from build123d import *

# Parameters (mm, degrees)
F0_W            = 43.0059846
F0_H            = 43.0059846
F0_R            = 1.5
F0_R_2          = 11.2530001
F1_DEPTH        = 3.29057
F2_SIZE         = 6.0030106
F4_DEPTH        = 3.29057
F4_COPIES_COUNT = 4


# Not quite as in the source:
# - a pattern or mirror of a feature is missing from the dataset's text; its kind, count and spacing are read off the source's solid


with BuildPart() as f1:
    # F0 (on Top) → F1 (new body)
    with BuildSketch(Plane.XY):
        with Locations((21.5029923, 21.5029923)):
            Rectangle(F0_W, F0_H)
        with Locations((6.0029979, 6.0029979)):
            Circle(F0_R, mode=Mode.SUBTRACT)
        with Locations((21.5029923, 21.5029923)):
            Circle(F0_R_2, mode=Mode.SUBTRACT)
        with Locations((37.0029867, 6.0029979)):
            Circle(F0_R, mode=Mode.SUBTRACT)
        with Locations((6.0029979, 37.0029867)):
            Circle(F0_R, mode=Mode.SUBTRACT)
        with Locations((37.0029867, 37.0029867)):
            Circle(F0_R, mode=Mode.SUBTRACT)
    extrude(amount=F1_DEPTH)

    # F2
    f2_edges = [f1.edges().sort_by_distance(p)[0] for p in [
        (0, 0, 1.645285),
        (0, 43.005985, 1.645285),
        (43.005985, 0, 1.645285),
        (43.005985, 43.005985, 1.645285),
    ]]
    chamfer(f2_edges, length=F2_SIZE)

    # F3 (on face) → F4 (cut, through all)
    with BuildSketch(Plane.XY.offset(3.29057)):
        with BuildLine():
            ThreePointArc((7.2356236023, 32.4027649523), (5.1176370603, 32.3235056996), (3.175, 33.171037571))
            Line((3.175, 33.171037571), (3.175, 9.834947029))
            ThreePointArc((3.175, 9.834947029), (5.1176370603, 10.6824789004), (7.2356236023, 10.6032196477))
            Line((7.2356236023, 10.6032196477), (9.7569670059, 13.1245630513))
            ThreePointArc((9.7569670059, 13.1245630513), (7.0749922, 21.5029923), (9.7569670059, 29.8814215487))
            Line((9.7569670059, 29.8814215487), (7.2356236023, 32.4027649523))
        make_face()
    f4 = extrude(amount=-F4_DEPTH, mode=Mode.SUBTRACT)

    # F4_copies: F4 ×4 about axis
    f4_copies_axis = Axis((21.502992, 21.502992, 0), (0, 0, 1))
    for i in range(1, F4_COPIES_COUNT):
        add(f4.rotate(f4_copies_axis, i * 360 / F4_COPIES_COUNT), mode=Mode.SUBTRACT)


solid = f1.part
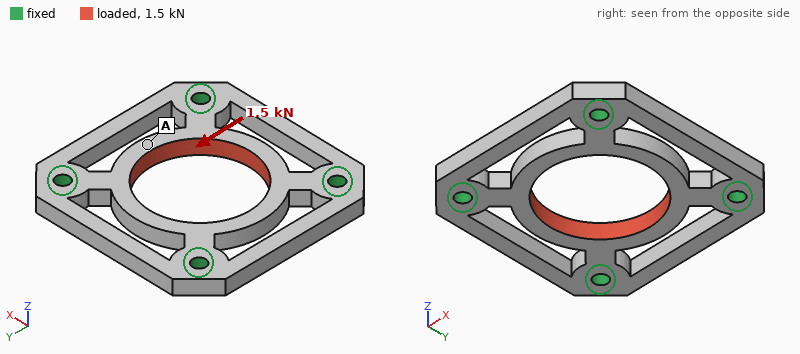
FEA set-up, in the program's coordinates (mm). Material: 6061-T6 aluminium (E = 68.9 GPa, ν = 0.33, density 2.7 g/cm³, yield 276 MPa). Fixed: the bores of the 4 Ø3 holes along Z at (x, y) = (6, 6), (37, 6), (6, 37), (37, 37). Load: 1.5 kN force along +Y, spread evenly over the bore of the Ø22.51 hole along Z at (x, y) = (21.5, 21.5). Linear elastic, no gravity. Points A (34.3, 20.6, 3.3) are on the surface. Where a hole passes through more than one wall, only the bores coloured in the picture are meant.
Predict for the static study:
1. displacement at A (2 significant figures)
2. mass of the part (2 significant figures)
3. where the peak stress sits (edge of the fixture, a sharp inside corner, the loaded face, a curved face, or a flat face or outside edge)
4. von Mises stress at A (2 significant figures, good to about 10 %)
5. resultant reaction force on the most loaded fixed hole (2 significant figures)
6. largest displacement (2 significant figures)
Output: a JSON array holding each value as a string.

["12 µm", "8.2 g", "edge of the fixture", "16 MPa", "380 N", "31 µm"]
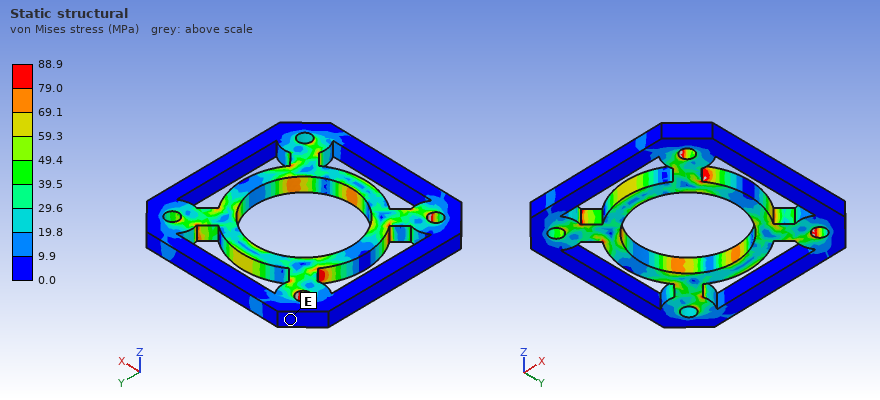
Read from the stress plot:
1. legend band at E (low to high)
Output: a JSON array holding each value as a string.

["0.0 to 9.9 MPa"]
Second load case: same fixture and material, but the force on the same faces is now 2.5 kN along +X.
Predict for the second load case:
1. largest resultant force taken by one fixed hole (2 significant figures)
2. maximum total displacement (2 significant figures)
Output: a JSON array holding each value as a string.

["630 N", "51 µm"]
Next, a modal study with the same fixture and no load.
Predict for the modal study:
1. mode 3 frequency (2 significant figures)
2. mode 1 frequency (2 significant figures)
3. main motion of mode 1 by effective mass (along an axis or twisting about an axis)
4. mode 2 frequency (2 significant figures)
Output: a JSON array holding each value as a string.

["18 kHz", "16 kHz", "along Z", "17 kHz"]
